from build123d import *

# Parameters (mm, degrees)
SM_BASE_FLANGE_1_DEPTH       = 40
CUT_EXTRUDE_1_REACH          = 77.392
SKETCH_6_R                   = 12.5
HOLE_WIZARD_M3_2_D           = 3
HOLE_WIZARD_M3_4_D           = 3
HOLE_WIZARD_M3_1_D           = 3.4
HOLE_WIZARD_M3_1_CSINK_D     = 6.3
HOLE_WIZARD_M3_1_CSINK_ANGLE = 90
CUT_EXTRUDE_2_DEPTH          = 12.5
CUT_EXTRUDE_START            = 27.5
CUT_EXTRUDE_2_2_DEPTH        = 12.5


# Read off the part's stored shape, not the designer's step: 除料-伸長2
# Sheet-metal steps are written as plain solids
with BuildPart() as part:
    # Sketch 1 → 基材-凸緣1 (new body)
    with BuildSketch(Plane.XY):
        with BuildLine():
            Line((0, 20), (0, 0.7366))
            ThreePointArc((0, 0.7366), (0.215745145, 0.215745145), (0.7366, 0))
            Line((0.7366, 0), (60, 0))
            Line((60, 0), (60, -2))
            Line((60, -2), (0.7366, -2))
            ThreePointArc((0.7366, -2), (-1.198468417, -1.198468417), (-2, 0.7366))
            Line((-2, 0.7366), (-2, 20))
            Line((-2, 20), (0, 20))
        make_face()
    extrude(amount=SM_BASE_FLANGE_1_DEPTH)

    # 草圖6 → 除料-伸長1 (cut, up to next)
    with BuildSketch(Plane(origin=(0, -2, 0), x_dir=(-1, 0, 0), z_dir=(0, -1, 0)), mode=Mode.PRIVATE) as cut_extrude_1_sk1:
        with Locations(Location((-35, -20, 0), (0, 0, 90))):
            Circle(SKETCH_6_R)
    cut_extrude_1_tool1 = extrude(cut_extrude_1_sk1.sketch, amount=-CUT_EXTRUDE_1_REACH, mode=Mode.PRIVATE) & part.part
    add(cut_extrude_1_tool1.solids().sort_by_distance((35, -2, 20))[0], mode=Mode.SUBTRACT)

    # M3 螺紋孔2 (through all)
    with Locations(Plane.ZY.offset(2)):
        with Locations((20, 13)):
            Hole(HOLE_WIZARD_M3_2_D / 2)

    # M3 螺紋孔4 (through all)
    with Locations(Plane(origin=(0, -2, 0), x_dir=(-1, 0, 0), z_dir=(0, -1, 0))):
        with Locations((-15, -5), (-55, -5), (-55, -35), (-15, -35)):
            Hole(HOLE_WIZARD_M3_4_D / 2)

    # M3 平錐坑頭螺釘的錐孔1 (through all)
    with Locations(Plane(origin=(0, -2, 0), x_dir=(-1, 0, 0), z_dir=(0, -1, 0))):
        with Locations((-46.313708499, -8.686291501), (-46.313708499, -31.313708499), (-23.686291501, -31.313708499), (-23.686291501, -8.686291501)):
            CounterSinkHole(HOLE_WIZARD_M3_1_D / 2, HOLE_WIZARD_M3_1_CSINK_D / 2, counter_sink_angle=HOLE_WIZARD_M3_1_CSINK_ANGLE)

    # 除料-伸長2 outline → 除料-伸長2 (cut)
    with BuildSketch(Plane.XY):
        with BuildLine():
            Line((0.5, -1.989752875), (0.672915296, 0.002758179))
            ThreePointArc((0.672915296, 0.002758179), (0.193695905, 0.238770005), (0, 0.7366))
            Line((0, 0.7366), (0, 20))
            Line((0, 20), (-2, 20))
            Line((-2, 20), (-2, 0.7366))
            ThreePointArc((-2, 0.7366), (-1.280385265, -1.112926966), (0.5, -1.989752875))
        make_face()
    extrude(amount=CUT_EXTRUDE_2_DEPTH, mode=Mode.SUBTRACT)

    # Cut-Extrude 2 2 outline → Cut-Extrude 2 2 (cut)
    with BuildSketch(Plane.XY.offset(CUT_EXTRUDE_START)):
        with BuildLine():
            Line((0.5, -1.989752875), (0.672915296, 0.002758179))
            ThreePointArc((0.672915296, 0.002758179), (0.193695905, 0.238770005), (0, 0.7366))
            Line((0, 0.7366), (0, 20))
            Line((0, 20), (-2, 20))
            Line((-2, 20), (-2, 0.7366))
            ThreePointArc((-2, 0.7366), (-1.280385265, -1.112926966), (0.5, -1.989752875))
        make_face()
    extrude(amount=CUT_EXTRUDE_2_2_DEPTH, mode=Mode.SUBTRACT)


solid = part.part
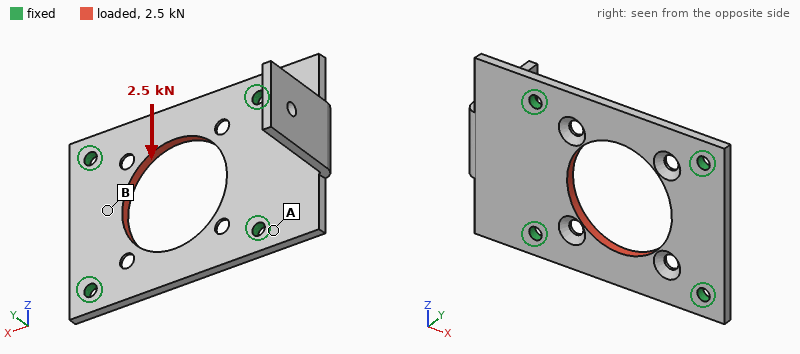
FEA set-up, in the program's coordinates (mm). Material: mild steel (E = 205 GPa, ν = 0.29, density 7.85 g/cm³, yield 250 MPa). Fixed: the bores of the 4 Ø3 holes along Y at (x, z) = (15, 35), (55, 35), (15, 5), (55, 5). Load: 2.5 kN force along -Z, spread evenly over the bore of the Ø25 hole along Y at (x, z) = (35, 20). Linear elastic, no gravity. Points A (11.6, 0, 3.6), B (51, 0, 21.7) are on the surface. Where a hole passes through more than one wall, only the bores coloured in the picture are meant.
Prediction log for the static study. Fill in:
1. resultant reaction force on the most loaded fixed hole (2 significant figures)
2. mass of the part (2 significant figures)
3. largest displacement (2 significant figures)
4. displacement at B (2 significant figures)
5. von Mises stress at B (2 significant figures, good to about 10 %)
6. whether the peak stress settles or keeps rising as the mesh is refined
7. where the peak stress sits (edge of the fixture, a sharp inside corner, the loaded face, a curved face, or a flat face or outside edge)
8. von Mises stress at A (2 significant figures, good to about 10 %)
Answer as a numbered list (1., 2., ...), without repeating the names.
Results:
1. 670 N
2. 33 g
3. 7.8 µm
4. 1.9 µm
5. 42 MPa
6. keeps rising
7. a sharp inside corner
8. 18 MPa
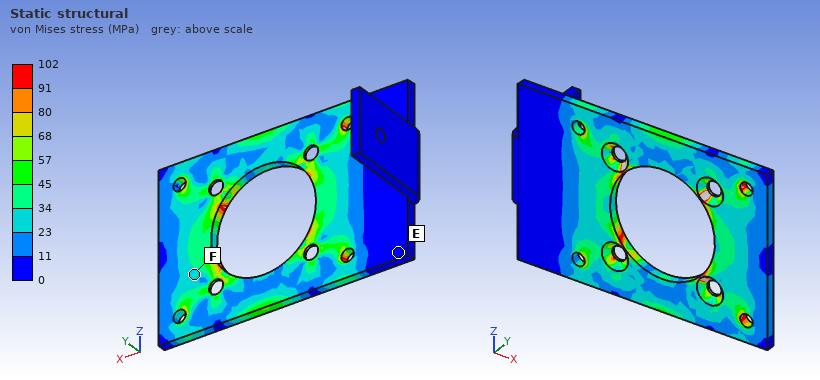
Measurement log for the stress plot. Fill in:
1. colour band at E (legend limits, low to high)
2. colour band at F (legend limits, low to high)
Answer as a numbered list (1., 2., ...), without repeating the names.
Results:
1. 0 to 11 MPa
2. 23 to 34 MPa
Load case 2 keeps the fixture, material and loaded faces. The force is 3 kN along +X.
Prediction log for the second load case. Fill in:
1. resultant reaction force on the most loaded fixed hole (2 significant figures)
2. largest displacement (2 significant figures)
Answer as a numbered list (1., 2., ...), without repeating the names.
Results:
1. 770 N
2. 4.1 µm
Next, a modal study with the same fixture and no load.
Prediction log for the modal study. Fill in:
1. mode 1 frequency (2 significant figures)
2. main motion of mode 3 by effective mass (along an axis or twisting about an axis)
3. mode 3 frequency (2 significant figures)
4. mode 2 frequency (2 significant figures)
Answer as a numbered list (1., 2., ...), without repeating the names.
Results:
1. 2100 Hz
2. along Y
3. 4500 Hz
4. 4100 Hz
